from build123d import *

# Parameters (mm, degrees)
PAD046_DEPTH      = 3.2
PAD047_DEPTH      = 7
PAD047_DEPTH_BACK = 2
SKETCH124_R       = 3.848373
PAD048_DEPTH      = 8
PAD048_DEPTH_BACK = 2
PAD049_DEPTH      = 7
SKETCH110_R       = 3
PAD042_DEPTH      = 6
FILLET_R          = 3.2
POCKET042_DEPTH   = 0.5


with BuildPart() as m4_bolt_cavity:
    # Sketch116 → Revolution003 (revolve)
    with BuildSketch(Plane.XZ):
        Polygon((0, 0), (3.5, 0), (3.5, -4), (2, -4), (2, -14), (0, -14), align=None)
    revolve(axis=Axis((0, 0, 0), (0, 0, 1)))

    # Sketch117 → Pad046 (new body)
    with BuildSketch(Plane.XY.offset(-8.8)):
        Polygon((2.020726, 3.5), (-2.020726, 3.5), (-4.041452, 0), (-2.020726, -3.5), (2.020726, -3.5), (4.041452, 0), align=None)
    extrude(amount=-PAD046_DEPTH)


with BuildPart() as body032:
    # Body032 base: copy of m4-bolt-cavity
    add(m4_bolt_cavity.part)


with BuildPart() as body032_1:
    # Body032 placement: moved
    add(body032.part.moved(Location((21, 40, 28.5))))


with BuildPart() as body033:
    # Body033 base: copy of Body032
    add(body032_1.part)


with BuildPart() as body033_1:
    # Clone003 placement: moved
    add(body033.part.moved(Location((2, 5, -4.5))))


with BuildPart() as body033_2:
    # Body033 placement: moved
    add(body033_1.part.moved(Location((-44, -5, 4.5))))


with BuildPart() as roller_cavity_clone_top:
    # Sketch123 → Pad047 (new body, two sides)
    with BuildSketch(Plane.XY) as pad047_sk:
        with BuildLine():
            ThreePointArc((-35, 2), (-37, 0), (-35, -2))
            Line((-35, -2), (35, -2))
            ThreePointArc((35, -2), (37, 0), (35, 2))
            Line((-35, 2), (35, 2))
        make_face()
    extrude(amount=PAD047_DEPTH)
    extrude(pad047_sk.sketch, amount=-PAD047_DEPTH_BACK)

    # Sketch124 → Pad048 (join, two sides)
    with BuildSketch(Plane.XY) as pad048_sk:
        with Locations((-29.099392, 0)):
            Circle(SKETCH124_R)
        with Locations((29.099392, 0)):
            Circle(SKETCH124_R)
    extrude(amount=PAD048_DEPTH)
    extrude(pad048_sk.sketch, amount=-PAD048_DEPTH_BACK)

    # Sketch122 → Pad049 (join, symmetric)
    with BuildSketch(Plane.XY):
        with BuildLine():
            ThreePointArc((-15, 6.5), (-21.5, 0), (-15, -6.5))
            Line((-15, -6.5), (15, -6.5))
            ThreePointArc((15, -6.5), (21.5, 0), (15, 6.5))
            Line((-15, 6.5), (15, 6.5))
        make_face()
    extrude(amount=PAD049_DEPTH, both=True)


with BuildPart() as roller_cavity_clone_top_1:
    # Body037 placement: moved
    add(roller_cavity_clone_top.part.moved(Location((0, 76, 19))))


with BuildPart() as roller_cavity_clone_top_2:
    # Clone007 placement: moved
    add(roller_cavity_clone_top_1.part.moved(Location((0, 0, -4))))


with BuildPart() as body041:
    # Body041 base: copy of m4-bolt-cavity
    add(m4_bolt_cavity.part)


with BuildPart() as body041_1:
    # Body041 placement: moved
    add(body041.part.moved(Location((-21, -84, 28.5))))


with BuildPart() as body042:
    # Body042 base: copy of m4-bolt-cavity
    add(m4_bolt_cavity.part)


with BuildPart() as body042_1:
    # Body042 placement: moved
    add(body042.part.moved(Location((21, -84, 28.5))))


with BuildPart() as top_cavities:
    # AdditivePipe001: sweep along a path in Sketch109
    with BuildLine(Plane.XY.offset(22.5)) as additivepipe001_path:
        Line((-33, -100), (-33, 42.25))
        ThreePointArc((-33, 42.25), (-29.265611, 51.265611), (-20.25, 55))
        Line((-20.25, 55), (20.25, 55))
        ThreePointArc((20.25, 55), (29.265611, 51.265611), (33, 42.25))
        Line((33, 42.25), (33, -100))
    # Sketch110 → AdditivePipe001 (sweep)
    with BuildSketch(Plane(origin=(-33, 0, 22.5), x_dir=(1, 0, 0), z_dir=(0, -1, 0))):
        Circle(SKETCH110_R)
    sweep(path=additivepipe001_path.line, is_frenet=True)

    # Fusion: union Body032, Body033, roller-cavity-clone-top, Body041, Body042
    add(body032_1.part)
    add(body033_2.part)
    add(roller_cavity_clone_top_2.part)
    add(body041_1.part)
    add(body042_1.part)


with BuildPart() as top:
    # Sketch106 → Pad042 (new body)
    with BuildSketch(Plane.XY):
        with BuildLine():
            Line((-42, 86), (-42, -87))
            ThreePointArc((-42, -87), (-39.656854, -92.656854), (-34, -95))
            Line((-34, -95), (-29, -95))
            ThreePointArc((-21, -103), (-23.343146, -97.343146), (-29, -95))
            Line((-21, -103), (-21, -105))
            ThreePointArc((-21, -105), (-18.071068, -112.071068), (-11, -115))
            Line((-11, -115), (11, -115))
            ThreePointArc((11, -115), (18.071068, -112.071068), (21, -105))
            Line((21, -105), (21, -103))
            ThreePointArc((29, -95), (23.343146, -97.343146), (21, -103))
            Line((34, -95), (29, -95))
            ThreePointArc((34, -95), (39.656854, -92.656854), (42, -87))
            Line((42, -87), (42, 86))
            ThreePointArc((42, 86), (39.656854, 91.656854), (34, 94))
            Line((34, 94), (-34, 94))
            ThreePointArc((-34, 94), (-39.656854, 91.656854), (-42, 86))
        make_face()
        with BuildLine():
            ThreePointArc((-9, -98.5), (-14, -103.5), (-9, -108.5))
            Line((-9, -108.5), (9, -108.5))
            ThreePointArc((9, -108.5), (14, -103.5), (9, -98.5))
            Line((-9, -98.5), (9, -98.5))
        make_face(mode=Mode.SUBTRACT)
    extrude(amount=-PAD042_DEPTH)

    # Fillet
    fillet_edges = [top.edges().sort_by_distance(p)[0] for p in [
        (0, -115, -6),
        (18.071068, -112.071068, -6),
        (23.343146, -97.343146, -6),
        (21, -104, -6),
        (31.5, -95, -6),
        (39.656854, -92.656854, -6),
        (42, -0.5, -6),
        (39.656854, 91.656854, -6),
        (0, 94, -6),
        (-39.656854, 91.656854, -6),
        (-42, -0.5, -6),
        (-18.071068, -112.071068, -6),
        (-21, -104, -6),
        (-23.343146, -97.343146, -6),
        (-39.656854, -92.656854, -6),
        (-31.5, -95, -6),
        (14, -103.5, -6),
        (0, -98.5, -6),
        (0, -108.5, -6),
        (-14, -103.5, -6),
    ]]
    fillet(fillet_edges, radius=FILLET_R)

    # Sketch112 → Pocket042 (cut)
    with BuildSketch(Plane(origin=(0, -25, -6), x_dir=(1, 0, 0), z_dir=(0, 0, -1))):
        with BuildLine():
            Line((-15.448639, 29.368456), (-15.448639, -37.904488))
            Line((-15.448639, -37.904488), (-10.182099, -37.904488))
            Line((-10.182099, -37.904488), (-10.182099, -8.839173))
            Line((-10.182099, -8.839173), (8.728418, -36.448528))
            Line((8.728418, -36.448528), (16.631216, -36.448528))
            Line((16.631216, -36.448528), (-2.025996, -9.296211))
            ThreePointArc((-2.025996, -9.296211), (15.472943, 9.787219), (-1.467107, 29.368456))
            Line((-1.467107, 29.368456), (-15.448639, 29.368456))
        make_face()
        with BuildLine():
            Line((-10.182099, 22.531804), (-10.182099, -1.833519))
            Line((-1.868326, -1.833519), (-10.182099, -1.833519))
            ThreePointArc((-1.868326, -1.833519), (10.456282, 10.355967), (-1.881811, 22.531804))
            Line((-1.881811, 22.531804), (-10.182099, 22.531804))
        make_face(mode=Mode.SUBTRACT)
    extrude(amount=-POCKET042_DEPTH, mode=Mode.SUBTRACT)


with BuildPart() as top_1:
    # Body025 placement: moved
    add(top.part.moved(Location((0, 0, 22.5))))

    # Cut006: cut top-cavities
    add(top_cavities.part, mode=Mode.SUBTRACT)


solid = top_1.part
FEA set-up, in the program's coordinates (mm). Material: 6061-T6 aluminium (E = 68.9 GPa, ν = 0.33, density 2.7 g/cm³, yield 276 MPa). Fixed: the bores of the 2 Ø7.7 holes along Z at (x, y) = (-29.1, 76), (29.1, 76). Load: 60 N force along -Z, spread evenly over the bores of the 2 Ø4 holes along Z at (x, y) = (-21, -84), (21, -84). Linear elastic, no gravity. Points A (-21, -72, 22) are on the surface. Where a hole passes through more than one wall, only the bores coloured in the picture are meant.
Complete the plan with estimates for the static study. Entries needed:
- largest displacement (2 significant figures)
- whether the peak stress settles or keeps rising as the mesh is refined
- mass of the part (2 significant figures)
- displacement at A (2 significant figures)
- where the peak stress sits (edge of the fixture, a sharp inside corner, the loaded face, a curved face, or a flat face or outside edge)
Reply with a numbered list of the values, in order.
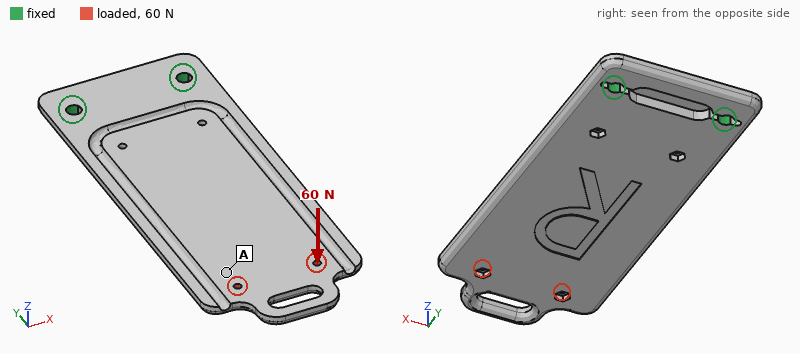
1. 1.5 mm
2. keeps rising
3. 230 g
4. 1.0 mm
5. edge of the fixture
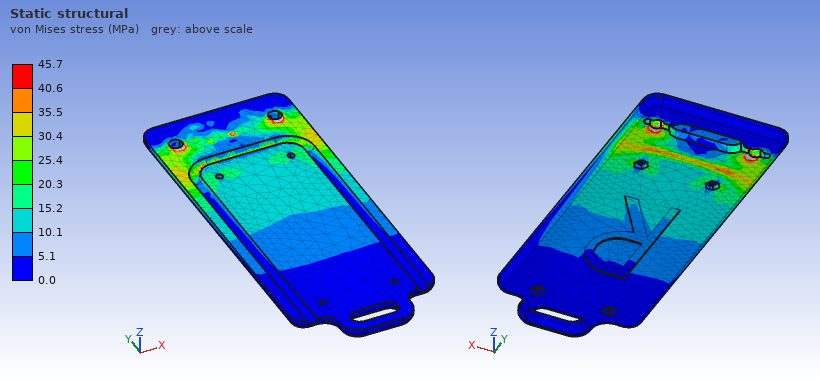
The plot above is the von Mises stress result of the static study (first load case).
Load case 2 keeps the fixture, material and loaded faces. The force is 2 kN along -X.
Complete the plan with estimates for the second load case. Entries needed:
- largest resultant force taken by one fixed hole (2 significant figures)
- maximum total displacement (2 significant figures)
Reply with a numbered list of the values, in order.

1. 5.3 kN
2. 0.30 mm
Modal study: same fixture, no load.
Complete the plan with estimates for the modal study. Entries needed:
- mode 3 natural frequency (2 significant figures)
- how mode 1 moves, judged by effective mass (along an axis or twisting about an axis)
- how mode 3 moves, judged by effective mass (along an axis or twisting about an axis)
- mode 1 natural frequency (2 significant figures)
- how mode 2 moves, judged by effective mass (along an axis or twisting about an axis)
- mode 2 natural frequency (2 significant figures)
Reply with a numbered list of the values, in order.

1. 890 Hz
2. along Z
3. along Z
4. 130 Hz
5. twisting about Y
6. 690 Hz
